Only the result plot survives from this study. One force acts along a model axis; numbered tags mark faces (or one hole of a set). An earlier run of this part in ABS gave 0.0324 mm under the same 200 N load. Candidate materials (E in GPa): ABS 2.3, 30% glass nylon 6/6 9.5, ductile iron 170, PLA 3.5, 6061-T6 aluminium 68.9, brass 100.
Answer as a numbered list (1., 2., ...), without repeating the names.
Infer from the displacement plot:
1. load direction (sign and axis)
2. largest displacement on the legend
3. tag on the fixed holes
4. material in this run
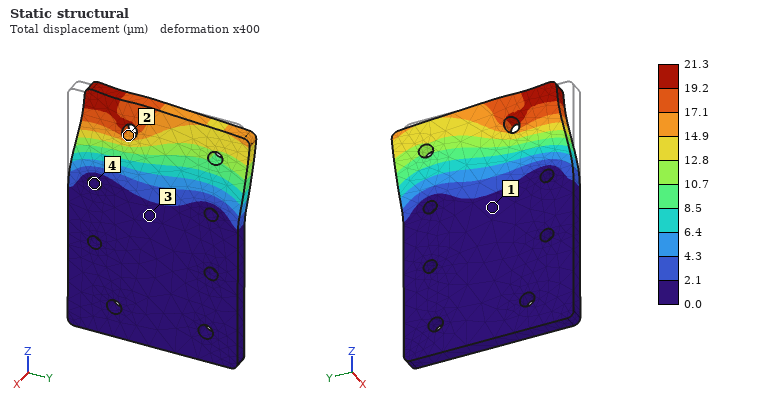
1. +Y
2. 21.3 µm
3. 4
4. PLA
